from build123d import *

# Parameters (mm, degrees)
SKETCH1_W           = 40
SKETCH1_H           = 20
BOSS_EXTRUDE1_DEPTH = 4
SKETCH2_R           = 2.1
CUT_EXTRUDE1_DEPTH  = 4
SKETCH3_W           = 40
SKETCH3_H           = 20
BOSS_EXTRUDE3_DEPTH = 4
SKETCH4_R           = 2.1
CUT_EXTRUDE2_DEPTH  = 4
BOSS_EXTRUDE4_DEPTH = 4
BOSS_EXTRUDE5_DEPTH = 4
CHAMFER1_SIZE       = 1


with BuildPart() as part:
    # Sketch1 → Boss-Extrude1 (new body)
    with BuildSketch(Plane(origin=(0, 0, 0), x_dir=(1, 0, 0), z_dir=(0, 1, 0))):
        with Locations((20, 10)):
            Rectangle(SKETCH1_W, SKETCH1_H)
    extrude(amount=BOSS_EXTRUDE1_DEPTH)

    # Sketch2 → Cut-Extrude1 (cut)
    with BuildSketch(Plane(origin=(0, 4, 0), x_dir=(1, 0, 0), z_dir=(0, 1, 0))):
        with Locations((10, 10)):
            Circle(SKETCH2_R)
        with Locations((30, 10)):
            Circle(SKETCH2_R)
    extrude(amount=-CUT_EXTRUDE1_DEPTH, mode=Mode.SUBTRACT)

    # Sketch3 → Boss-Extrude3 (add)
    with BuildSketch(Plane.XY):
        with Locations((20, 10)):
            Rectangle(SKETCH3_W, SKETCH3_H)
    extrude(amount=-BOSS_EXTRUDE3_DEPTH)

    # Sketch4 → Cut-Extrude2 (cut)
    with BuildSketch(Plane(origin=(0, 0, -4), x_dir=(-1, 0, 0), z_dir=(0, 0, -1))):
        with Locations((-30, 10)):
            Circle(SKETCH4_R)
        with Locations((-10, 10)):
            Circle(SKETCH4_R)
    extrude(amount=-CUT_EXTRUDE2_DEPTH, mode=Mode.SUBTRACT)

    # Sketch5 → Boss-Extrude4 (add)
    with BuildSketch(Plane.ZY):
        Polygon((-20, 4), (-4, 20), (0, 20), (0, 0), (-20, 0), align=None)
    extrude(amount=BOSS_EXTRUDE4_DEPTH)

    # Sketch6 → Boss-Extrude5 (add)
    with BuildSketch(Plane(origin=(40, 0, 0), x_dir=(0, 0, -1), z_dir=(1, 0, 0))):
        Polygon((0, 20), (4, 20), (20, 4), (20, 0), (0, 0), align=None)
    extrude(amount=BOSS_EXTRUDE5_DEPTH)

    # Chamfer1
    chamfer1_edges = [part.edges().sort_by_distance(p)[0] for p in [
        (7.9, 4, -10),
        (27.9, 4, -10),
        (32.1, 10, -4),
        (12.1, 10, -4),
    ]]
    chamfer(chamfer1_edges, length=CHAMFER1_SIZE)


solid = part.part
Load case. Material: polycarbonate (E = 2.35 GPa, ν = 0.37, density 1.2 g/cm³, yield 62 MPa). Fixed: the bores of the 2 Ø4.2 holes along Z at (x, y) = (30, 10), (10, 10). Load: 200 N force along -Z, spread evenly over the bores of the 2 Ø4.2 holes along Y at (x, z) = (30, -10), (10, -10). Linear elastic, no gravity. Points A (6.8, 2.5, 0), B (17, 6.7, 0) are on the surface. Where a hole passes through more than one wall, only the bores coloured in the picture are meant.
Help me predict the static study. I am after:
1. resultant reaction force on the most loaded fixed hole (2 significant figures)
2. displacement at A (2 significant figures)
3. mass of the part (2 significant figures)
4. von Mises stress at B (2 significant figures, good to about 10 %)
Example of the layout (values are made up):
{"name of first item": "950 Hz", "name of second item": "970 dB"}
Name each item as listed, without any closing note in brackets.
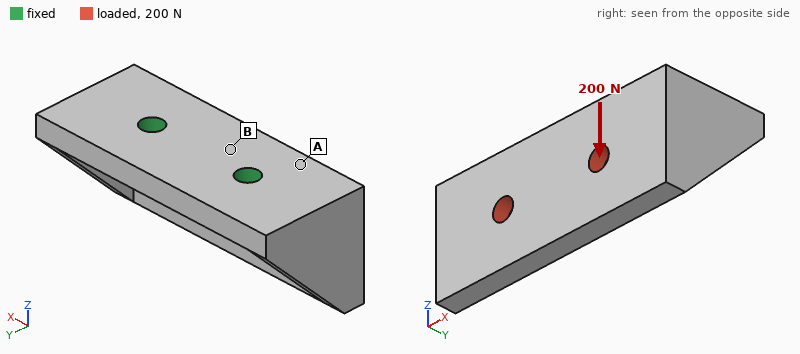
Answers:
{"resultant reaction force on the most loaded fixed hole": "100 N", "displacement at A": "0.096 mm", "mass of the part": "9.2 g", "von Mises stress at B": "4.5 MPa"}
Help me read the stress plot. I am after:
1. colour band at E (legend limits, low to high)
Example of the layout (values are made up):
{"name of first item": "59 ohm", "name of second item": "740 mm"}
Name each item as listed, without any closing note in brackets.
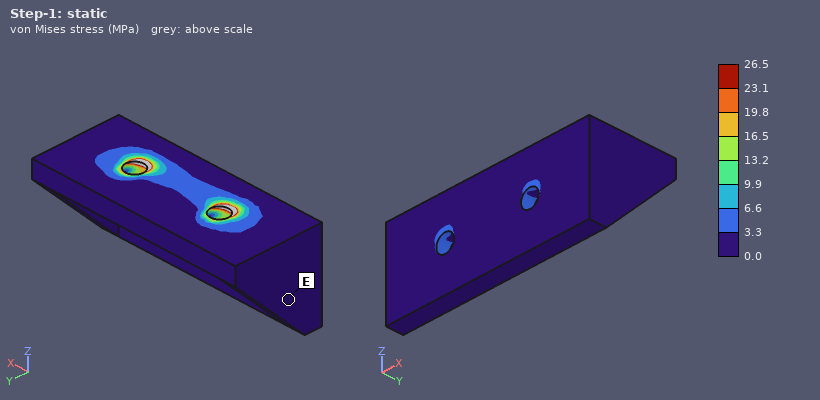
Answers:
{"colour band at E": "0.0 to 3.3 MPa"}
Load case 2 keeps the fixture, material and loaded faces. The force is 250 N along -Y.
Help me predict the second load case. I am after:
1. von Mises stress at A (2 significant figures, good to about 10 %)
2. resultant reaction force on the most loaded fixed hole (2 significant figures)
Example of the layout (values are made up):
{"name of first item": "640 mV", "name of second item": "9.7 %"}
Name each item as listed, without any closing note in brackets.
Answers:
{"von Mises stress at A": "4.4 MPa", "resultant reaction force on the most loaded fixed hole": "130 N"}
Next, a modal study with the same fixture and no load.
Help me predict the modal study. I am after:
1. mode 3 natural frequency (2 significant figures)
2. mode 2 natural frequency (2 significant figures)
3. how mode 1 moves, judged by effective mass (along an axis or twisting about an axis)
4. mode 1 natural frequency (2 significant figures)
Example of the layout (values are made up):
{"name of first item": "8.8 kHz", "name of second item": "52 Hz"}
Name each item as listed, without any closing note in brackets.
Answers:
{"mode 3 natural frequency": "3200 Hz", "mode 2 natural frequency": "2100 Hz", "how mode 1 moves, judged by effective mass": "along Y", "mode 1 natural frequency": "1700 Hz"}
